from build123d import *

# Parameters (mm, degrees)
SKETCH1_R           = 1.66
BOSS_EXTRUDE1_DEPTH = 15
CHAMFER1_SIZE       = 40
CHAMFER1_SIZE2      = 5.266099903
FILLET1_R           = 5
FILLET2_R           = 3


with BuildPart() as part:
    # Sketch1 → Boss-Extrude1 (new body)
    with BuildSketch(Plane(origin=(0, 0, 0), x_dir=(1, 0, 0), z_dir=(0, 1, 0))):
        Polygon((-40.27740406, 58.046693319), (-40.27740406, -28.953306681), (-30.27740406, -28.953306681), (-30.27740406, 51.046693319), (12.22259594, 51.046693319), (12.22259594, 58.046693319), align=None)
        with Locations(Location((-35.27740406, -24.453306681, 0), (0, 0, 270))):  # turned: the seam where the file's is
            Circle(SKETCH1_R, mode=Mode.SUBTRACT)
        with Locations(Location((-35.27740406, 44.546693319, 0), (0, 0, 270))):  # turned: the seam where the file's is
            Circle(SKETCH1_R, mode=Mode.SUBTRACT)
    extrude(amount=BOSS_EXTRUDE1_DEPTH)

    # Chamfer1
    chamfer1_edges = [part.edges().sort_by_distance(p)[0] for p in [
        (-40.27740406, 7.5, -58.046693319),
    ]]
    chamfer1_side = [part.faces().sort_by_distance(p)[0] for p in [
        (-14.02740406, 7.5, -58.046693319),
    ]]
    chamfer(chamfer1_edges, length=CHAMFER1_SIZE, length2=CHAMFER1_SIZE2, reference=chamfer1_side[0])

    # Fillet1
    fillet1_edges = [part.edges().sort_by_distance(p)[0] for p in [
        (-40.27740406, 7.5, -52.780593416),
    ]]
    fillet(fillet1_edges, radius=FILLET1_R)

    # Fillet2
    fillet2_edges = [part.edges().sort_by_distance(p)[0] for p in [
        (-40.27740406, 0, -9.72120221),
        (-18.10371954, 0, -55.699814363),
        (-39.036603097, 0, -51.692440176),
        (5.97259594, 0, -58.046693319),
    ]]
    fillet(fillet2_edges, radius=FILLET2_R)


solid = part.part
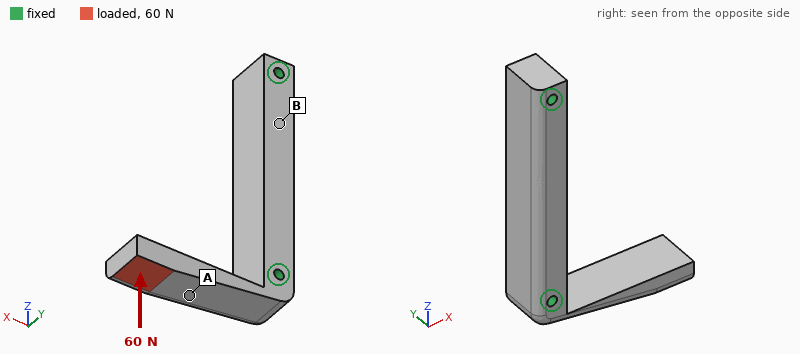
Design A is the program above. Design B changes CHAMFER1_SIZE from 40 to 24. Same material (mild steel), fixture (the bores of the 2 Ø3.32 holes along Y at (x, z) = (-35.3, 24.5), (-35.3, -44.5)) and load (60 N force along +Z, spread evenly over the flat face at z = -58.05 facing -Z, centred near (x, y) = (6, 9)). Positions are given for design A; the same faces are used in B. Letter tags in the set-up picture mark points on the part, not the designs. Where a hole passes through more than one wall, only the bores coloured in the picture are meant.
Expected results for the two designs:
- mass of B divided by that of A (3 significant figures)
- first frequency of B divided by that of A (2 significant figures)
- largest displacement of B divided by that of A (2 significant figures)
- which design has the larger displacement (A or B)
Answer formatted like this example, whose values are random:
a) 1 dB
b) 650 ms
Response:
a) 1.04
b) 1.4
c) 0.38
d) A
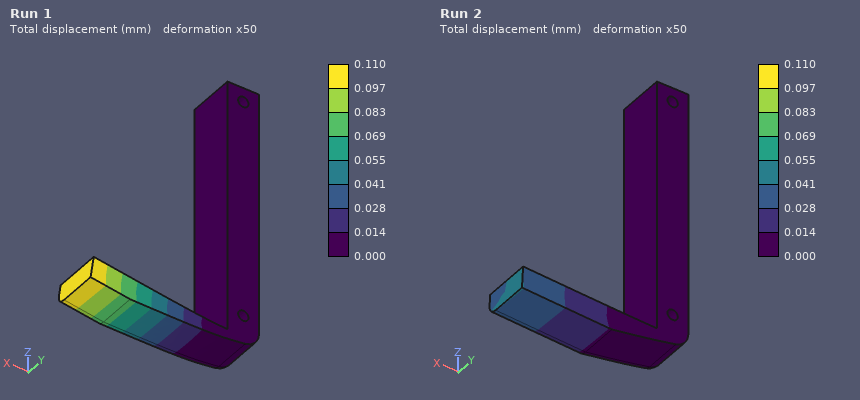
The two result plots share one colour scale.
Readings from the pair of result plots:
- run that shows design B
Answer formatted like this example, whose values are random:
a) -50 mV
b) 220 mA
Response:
a) Run 2
